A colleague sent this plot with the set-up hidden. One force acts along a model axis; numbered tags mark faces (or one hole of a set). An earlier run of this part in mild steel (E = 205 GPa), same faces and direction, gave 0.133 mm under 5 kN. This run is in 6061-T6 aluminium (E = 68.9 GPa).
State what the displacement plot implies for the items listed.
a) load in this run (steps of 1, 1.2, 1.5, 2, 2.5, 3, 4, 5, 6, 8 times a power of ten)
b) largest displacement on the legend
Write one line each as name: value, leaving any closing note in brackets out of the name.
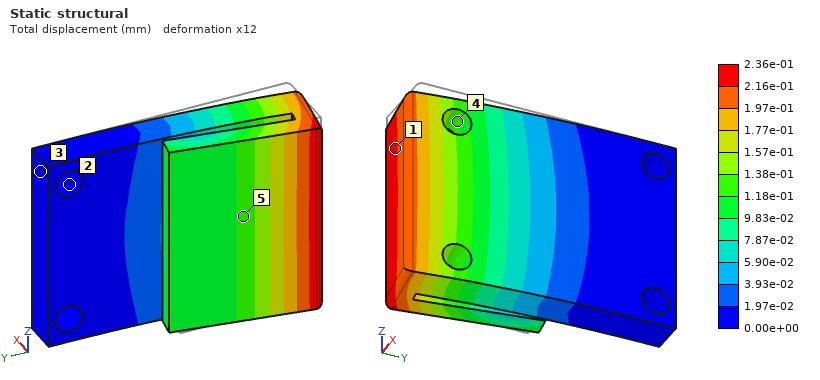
load in this run: 3 kN
largest displacement on the legend: 2.36e-01 mm
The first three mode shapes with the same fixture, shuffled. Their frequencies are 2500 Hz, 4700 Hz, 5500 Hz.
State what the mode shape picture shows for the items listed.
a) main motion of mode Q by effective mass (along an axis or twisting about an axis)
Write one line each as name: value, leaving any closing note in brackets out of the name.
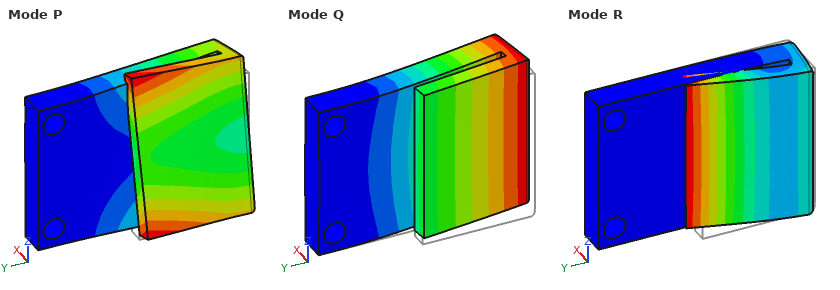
main motion of mode Q by effective mass: along X
